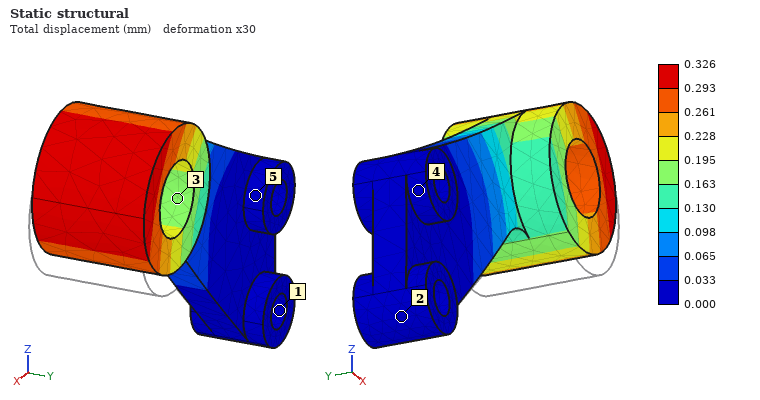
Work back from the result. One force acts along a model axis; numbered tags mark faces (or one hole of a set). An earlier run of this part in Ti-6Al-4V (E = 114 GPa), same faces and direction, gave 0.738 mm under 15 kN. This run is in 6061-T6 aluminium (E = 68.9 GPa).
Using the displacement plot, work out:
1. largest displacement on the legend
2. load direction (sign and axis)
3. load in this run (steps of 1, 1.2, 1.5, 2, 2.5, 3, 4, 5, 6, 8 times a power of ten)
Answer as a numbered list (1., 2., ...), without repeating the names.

1. 0.326 mm
2. +Z
3. 4 kN
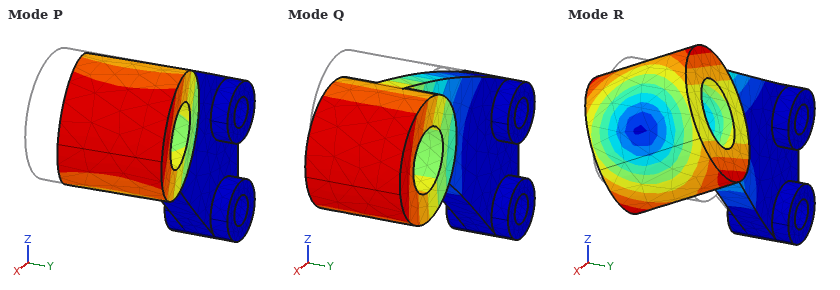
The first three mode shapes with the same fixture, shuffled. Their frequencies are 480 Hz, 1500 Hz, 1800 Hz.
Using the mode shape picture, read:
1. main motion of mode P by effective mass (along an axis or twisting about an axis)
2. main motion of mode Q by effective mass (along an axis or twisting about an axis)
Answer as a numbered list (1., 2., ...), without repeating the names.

1. along Y
2. along Z
